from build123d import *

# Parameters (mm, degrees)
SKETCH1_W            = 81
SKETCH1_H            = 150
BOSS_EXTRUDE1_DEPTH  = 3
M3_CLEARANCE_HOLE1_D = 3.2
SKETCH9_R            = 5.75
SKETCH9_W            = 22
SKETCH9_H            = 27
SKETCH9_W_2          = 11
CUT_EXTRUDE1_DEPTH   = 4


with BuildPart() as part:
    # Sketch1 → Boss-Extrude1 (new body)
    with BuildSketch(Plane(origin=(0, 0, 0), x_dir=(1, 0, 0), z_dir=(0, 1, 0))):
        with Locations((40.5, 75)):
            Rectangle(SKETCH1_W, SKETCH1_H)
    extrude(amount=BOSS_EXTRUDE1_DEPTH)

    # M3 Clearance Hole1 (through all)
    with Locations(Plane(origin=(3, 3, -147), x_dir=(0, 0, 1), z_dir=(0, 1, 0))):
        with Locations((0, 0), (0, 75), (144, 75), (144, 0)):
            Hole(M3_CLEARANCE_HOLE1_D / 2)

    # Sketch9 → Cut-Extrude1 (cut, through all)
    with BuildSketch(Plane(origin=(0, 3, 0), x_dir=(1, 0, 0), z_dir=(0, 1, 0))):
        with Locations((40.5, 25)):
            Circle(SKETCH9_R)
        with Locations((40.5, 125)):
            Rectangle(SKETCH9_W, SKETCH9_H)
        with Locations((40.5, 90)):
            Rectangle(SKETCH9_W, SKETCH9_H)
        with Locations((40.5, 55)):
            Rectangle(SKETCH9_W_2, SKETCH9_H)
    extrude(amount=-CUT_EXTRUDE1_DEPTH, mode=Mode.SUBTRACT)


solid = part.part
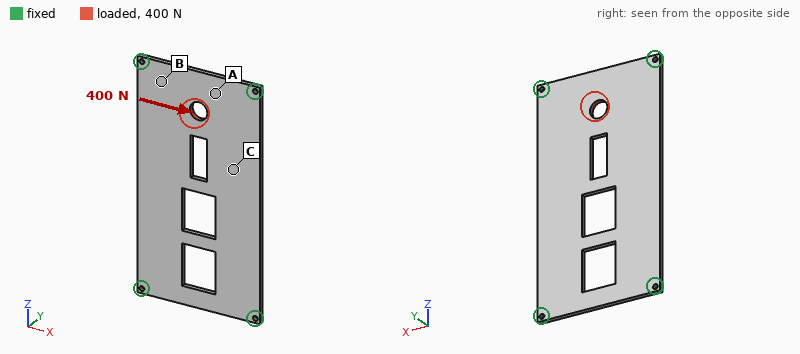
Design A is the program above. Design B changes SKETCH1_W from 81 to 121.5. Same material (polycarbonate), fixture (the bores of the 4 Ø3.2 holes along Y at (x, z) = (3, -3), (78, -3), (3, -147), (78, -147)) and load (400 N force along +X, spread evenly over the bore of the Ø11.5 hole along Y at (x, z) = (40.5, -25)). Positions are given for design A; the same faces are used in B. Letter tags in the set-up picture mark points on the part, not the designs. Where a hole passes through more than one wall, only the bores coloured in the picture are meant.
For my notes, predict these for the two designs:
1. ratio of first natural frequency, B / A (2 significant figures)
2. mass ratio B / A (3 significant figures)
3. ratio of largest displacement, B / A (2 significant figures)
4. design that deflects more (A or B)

1.0
1.58
0.77
A
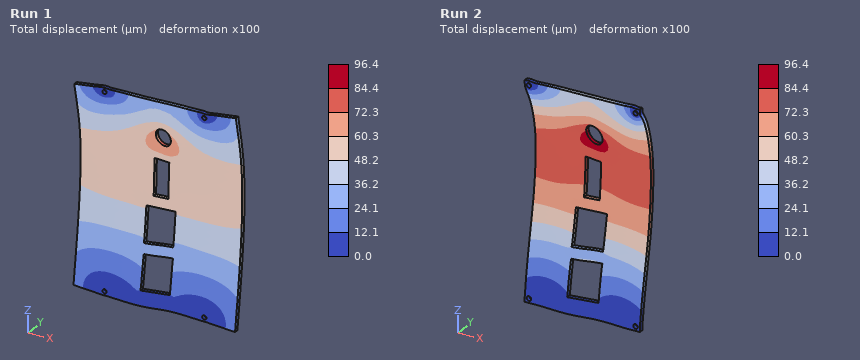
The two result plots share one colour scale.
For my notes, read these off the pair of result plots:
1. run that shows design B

Run 1
